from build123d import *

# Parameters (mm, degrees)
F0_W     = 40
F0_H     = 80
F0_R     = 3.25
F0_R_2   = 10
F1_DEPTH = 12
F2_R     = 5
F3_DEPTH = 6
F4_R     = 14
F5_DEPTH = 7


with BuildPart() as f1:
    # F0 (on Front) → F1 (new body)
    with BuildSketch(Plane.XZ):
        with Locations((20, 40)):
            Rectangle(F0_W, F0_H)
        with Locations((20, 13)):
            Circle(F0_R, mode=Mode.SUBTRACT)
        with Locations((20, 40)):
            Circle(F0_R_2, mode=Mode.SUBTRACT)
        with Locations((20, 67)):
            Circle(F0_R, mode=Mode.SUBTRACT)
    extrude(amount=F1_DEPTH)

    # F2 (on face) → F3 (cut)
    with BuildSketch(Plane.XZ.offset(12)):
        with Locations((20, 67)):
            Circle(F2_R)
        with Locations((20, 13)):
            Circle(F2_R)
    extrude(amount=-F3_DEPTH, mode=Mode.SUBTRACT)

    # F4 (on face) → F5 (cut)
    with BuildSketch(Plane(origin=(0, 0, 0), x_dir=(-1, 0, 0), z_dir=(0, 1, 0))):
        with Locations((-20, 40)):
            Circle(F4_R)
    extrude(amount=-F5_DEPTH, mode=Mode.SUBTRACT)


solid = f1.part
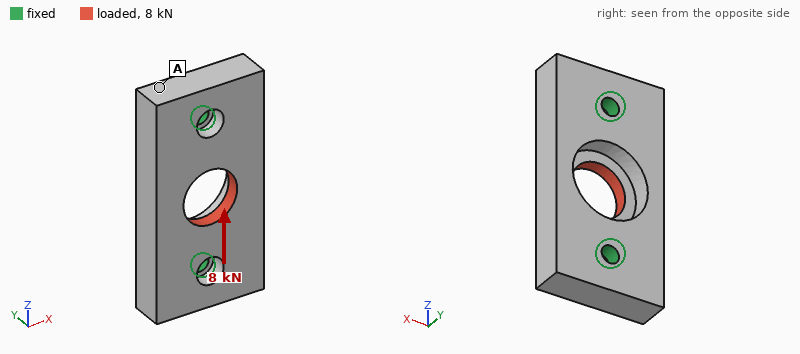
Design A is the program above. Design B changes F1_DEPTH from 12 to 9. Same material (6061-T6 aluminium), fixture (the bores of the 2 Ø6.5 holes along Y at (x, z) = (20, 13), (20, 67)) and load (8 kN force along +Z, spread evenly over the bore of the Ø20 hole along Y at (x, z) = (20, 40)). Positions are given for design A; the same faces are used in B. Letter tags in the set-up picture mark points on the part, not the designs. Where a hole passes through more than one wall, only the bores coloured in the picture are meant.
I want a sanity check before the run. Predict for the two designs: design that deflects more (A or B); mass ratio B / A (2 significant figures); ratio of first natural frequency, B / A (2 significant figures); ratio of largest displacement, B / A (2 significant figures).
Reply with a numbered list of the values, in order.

1. B
2. 0.74
3. 1.1
4. 1.6
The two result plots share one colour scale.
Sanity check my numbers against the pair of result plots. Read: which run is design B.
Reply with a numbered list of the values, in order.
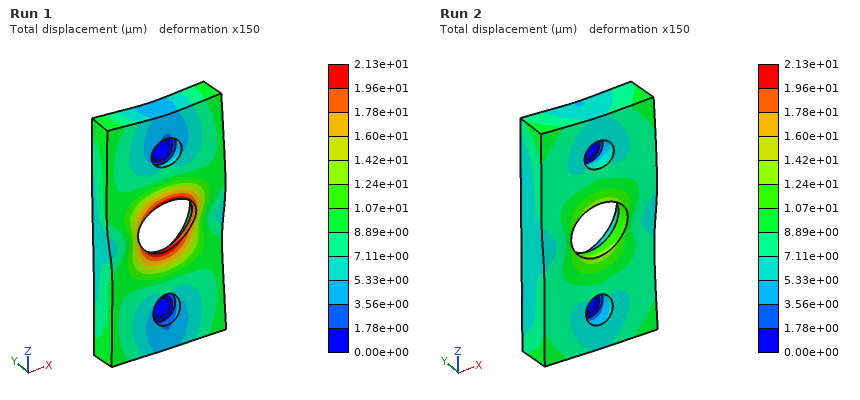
1. Run 1
